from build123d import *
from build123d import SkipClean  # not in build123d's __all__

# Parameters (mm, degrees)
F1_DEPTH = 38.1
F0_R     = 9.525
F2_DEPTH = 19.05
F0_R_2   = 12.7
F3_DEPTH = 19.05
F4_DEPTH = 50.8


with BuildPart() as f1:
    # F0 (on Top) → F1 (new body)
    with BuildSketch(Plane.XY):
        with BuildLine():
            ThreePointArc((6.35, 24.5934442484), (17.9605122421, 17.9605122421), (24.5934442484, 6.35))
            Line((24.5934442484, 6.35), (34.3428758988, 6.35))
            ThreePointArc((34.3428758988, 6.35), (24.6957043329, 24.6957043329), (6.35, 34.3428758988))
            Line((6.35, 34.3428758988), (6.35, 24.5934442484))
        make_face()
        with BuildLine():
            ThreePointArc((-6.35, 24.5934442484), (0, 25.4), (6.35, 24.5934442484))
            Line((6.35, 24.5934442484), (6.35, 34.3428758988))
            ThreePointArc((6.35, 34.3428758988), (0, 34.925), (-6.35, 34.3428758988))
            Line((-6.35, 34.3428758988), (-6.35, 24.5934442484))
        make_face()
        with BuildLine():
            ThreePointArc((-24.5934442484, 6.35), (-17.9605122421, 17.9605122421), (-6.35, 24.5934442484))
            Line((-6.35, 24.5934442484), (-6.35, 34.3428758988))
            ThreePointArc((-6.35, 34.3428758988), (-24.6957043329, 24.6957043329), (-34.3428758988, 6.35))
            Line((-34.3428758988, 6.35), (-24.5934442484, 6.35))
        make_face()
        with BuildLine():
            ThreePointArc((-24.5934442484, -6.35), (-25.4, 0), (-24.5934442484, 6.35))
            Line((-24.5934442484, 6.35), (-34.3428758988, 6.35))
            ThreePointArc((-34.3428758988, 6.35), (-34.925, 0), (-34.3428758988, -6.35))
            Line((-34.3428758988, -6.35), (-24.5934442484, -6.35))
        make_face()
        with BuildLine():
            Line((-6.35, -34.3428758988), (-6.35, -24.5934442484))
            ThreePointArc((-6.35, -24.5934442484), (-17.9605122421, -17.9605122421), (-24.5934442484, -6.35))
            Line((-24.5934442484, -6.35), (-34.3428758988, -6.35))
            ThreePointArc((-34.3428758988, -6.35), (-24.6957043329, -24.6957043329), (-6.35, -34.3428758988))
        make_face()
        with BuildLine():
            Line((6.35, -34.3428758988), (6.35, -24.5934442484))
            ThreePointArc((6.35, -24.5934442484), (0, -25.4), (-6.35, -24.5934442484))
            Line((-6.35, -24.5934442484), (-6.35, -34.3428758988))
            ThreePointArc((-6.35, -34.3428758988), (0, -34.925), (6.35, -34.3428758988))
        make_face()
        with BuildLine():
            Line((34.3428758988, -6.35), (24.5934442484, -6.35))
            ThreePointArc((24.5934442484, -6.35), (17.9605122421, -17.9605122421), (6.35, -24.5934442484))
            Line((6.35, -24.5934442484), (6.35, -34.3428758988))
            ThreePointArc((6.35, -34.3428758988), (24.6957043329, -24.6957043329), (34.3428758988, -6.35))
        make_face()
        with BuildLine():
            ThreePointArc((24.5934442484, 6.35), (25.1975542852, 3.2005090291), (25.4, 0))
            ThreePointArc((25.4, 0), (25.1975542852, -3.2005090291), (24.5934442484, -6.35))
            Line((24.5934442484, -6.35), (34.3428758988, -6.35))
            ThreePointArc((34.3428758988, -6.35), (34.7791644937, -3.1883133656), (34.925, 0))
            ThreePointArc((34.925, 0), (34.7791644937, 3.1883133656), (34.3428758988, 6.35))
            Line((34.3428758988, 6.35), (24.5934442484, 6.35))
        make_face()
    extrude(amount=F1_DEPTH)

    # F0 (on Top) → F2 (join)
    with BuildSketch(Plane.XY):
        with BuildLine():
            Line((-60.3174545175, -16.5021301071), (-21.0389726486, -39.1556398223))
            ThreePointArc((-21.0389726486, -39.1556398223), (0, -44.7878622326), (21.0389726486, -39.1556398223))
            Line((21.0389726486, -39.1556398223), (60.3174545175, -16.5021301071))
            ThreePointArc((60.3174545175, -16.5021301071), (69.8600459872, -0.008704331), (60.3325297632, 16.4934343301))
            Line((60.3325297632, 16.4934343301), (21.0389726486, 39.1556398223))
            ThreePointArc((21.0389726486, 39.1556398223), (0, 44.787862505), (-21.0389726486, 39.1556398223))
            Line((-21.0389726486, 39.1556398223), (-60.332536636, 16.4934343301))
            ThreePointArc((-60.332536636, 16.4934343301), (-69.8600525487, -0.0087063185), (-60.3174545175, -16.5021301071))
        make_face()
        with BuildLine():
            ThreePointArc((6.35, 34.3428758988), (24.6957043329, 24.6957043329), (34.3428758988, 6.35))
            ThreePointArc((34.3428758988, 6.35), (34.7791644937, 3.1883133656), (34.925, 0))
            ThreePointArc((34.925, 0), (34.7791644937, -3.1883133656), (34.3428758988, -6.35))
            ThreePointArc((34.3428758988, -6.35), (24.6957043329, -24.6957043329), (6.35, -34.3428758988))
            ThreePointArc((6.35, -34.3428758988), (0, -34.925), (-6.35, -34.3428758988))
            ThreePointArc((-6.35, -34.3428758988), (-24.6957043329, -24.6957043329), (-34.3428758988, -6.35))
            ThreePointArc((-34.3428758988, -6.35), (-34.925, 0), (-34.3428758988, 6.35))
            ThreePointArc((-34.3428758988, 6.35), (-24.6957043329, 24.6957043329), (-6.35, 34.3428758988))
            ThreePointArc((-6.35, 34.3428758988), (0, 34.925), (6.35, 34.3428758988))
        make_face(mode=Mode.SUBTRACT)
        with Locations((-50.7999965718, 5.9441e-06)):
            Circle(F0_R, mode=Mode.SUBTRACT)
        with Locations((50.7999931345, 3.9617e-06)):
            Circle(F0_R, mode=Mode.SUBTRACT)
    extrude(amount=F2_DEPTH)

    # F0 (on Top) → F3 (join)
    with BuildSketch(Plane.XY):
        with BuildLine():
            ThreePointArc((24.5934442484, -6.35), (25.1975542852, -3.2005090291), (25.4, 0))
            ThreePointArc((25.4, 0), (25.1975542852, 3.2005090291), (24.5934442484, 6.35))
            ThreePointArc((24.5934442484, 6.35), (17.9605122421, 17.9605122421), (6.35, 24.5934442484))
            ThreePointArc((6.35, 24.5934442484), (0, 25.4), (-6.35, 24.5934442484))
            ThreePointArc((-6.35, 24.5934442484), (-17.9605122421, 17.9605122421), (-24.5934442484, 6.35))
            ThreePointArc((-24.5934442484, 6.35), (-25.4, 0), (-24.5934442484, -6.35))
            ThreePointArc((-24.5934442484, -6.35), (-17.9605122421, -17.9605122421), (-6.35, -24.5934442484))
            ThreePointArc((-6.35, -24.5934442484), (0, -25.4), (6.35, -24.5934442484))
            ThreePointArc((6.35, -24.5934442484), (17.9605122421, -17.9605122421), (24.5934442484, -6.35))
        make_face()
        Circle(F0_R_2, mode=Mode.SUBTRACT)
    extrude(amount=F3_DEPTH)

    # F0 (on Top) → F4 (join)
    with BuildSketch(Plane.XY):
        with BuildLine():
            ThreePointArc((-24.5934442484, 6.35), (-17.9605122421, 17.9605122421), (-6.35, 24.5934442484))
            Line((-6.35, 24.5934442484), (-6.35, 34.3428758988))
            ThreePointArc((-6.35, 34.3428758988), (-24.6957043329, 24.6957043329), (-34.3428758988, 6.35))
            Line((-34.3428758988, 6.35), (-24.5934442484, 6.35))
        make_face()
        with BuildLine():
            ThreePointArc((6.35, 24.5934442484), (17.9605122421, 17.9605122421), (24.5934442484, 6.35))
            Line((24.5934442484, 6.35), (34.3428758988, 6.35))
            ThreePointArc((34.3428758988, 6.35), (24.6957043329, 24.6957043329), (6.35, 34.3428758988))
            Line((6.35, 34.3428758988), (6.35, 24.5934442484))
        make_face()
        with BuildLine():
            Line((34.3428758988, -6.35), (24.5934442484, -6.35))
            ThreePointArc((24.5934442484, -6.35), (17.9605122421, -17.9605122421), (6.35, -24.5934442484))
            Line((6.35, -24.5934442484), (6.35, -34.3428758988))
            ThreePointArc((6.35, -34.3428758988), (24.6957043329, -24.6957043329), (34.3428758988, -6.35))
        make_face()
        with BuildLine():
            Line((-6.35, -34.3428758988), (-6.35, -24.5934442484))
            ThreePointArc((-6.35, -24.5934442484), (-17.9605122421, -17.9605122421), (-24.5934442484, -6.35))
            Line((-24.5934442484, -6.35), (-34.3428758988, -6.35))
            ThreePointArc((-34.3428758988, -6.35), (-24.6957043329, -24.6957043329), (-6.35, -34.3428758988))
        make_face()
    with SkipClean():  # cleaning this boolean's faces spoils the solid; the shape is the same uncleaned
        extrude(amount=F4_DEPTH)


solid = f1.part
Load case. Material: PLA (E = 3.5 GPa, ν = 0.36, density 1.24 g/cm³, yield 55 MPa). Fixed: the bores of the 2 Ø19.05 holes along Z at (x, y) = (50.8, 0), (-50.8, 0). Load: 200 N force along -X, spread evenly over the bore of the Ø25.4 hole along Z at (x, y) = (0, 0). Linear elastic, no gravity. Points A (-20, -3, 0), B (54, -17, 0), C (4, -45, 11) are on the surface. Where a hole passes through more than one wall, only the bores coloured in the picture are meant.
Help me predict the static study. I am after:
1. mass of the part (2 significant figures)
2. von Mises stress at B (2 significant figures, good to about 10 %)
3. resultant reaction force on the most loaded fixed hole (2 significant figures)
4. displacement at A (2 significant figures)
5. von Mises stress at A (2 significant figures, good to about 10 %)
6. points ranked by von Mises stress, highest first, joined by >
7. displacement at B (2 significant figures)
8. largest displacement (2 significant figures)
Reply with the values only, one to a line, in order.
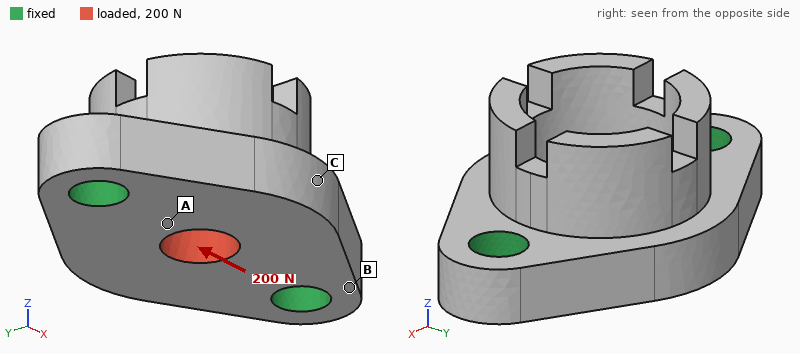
240 g
0.049 MPa
100 N
1.0 µm
0.16 MPa
A > B > C
0.28 µm
1.6 µm
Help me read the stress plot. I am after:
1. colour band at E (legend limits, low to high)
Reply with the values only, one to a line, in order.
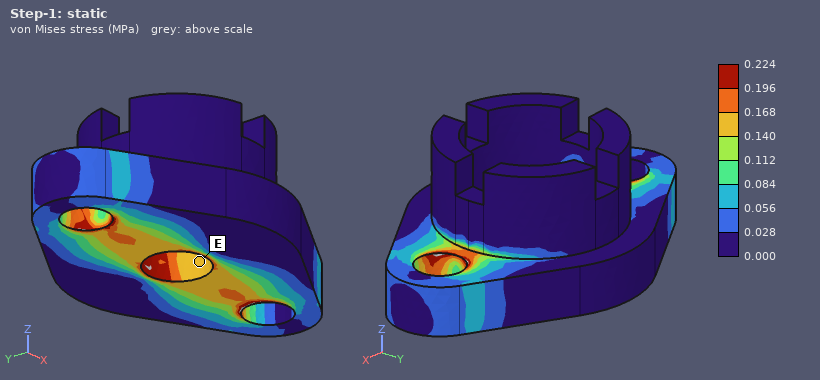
0.140 to 0.168 MPa
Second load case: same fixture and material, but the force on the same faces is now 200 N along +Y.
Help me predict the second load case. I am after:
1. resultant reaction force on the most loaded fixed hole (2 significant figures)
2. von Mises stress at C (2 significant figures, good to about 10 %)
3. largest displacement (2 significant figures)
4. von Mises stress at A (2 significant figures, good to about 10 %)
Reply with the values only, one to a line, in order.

100 N
0.10 MPa
3.4 µm
0.12 MPa
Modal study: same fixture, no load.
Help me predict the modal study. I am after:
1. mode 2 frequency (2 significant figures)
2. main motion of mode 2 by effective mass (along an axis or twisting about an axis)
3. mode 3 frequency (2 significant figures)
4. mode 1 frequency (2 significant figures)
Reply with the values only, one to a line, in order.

2100 Hz
along Z
2900 Hz
1600 Hz
